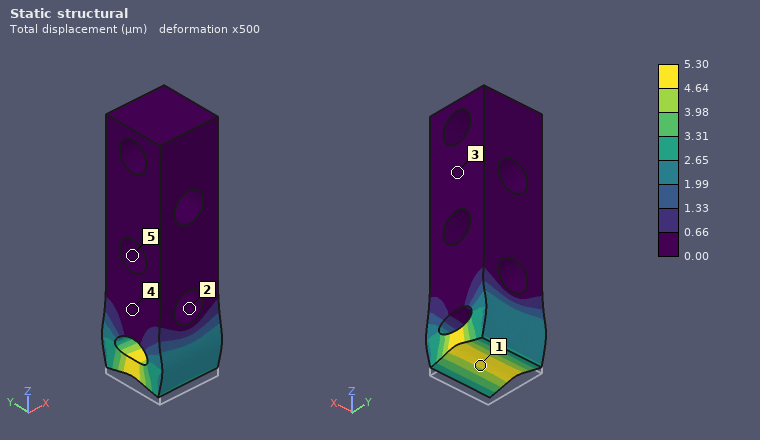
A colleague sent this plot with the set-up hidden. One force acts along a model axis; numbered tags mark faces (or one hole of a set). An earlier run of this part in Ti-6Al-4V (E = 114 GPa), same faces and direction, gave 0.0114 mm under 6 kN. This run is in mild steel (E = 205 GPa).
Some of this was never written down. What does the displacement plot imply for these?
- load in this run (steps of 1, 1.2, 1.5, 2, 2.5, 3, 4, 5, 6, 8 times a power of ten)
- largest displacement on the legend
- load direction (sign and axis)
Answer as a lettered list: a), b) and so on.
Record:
a) 5 kN
b) 5.30 µm
c) +Z
